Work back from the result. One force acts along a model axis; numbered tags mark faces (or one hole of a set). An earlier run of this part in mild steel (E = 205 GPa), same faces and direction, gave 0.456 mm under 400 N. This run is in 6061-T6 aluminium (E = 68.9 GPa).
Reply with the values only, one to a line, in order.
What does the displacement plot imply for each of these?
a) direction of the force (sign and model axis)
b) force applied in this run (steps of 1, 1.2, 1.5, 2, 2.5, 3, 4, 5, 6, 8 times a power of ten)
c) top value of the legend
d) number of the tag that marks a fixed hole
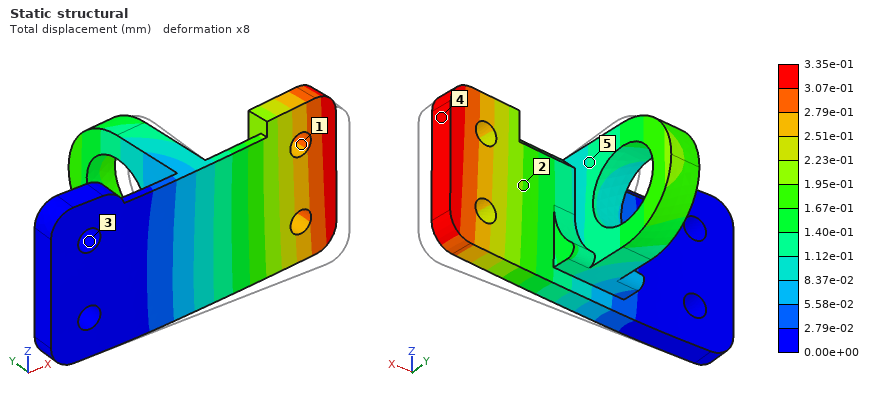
+Y
100 N
3.35e-01 mm
3
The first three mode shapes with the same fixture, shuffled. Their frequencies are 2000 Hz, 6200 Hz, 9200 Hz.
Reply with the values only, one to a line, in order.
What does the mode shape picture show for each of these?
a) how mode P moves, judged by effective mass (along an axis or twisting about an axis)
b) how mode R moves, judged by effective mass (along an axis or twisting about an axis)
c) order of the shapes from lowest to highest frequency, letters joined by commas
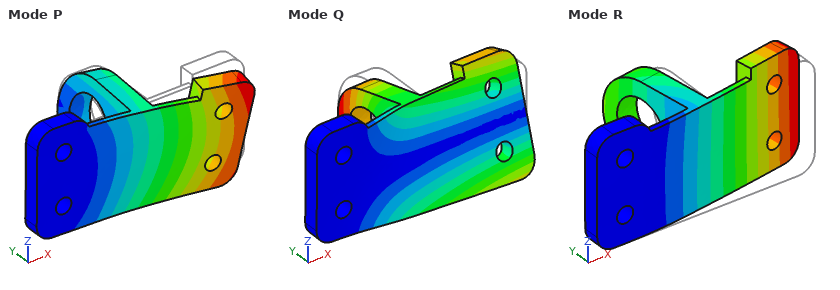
along Z
along Y
R, Q, P
